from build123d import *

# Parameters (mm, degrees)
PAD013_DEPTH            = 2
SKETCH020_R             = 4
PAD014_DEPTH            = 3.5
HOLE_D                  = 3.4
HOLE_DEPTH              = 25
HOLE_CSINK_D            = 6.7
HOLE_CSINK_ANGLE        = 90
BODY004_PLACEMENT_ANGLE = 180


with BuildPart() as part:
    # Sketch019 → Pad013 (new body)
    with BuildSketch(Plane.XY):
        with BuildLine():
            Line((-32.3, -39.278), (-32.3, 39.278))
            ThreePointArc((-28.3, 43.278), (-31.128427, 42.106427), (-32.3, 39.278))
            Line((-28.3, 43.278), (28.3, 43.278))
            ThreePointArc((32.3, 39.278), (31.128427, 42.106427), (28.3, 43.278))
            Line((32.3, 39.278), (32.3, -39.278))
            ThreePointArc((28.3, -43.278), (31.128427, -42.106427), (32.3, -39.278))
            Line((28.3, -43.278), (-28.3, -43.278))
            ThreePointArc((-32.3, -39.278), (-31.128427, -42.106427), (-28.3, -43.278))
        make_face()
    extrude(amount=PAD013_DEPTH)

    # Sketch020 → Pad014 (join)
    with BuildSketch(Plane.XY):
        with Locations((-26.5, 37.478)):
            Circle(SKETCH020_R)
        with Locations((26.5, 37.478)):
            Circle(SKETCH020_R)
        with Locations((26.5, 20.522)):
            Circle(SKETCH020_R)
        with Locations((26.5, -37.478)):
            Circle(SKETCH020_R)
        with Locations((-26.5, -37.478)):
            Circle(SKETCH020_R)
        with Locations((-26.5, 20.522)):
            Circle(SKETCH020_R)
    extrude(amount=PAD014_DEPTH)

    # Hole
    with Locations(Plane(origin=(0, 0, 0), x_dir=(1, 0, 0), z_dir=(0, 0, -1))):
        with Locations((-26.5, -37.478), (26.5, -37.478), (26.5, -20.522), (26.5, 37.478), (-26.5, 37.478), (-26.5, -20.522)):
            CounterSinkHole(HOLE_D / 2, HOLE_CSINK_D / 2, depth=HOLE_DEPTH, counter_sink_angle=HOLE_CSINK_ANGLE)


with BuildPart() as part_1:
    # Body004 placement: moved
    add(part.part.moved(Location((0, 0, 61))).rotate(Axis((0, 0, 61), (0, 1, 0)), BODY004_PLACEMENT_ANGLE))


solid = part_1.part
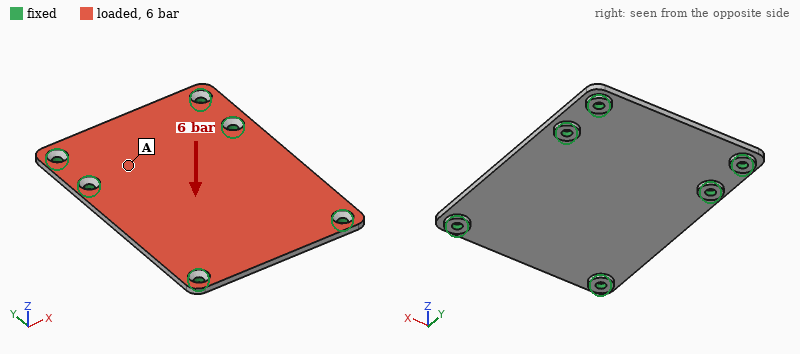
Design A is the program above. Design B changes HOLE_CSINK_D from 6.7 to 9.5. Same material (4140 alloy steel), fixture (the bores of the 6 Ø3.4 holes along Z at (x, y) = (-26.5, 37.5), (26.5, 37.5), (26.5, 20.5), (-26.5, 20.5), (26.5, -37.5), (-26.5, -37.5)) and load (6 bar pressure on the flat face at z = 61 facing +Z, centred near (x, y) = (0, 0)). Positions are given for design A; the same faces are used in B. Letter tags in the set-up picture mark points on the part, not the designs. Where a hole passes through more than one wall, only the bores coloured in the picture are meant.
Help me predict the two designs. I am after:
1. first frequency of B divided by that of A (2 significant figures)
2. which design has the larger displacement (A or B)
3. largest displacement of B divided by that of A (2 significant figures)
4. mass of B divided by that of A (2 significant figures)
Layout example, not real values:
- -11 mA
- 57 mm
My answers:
- 0.94
- B
- 1.1
- 0.97
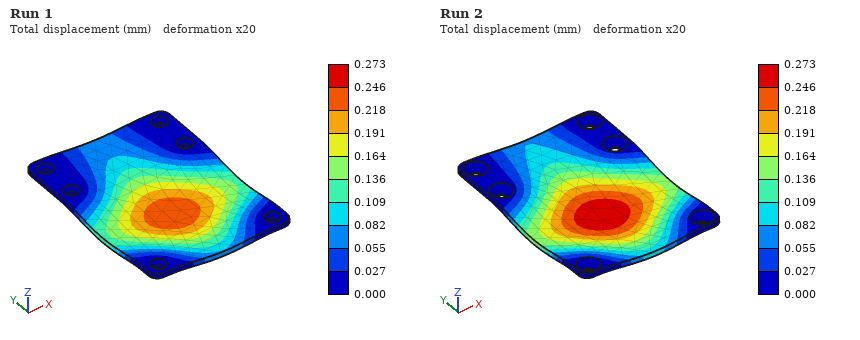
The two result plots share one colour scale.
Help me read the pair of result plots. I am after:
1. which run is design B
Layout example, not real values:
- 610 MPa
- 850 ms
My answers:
- Run 2
